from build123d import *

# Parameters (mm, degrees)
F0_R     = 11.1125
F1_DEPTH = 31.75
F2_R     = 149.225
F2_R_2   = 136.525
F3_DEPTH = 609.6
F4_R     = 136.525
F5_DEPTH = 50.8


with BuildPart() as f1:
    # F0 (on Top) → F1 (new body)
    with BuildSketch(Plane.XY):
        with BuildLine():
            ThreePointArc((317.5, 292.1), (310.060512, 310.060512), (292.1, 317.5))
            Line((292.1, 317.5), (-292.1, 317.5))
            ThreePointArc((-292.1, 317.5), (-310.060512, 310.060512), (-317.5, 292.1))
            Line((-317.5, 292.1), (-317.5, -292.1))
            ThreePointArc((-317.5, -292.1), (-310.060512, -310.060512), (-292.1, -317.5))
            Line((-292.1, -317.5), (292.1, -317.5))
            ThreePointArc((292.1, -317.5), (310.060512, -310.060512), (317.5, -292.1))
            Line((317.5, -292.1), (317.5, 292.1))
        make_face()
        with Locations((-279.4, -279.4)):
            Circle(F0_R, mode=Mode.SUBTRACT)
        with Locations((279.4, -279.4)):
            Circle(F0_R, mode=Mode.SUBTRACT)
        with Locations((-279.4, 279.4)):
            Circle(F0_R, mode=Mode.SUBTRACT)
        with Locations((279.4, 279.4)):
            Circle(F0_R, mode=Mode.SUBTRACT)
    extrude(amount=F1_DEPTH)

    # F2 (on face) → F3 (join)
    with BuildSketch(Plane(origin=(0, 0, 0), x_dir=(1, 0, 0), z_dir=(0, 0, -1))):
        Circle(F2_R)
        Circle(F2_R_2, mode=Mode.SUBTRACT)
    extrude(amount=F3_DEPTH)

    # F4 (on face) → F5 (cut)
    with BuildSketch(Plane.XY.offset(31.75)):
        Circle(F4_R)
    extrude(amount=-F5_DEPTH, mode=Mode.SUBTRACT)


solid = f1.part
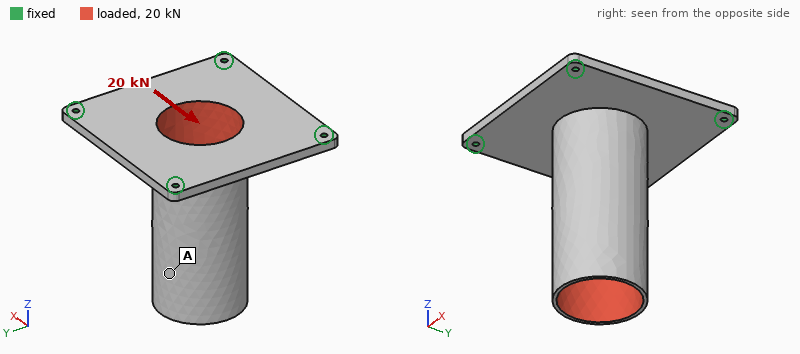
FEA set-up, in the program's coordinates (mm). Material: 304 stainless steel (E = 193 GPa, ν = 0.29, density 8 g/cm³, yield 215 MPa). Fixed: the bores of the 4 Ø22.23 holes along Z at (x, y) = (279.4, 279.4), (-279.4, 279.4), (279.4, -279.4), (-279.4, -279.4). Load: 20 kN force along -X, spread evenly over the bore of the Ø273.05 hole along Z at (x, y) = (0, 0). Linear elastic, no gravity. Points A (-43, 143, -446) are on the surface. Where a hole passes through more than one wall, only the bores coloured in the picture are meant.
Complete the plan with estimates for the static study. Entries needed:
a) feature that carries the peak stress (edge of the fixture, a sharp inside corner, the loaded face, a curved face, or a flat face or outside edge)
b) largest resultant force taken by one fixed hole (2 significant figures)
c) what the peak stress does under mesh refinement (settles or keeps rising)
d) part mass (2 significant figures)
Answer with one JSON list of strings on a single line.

["edge of the fixture", "8.9 kN", "keeps rising", "140 kg"]
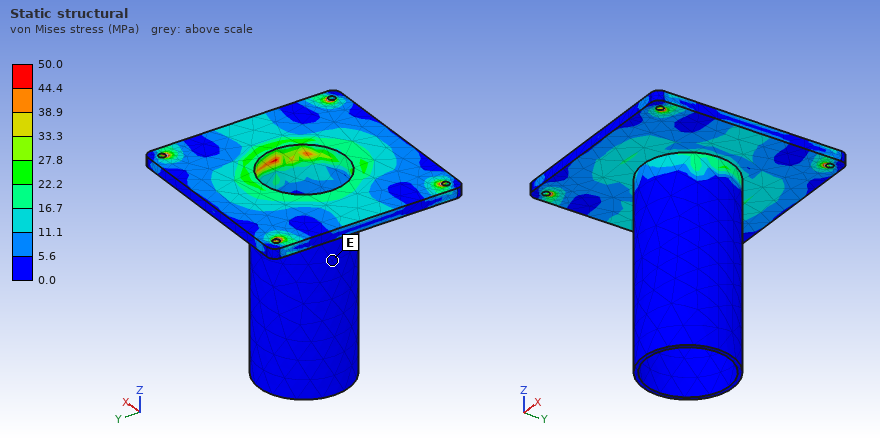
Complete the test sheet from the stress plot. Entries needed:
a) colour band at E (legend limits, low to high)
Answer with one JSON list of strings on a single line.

["0.0 to 5.6 MPa"]
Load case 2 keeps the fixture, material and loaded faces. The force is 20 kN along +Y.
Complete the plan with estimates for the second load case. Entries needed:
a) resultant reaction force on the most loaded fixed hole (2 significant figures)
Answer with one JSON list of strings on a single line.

["8.8 kN"]
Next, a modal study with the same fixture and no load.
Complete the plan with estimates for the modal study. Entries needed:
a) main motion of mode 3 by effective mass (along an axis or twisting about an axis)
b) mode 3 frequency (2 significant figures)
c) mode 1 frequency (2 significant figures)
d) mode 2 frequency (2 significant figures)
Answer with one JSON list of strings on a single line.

["along Z", "230 Hz", "150 Hz", "150 Hz"]
